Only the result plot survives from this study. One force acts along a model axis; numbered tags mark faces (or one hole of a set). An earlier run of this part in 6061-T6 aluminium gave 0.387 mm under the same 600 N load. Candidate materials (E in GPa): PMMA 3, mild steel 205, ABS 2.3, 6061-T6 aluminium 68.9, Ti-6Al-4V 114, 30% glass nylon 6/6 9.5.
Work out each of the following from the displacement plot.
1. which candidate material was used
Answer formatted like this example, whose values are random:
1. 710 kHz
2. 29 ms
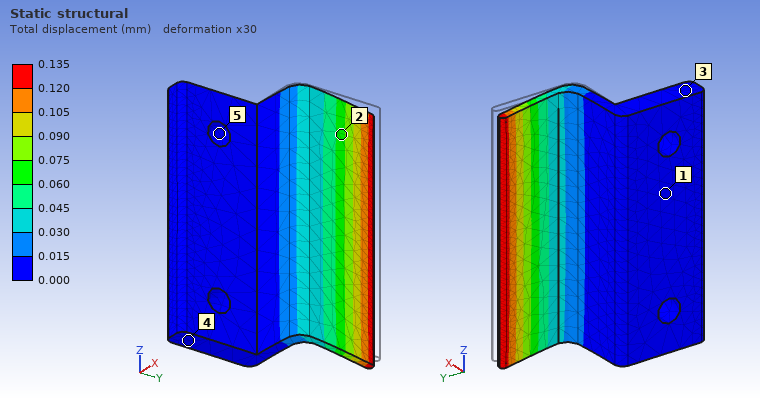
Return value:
1. mild steel
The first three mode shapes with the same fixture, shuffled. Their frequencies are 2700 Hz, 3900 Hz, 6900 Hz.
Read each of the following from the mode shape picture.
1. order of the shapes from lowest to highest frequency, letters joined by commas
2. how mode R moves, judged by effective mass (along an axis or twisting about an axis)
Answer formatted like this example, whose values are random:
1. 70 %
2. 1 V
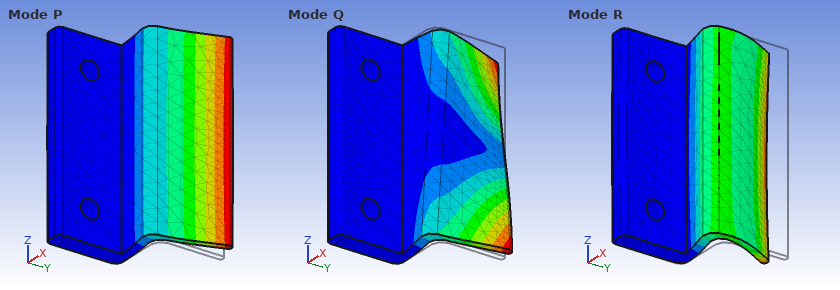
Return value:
1. P, Q, R
2. along Y
